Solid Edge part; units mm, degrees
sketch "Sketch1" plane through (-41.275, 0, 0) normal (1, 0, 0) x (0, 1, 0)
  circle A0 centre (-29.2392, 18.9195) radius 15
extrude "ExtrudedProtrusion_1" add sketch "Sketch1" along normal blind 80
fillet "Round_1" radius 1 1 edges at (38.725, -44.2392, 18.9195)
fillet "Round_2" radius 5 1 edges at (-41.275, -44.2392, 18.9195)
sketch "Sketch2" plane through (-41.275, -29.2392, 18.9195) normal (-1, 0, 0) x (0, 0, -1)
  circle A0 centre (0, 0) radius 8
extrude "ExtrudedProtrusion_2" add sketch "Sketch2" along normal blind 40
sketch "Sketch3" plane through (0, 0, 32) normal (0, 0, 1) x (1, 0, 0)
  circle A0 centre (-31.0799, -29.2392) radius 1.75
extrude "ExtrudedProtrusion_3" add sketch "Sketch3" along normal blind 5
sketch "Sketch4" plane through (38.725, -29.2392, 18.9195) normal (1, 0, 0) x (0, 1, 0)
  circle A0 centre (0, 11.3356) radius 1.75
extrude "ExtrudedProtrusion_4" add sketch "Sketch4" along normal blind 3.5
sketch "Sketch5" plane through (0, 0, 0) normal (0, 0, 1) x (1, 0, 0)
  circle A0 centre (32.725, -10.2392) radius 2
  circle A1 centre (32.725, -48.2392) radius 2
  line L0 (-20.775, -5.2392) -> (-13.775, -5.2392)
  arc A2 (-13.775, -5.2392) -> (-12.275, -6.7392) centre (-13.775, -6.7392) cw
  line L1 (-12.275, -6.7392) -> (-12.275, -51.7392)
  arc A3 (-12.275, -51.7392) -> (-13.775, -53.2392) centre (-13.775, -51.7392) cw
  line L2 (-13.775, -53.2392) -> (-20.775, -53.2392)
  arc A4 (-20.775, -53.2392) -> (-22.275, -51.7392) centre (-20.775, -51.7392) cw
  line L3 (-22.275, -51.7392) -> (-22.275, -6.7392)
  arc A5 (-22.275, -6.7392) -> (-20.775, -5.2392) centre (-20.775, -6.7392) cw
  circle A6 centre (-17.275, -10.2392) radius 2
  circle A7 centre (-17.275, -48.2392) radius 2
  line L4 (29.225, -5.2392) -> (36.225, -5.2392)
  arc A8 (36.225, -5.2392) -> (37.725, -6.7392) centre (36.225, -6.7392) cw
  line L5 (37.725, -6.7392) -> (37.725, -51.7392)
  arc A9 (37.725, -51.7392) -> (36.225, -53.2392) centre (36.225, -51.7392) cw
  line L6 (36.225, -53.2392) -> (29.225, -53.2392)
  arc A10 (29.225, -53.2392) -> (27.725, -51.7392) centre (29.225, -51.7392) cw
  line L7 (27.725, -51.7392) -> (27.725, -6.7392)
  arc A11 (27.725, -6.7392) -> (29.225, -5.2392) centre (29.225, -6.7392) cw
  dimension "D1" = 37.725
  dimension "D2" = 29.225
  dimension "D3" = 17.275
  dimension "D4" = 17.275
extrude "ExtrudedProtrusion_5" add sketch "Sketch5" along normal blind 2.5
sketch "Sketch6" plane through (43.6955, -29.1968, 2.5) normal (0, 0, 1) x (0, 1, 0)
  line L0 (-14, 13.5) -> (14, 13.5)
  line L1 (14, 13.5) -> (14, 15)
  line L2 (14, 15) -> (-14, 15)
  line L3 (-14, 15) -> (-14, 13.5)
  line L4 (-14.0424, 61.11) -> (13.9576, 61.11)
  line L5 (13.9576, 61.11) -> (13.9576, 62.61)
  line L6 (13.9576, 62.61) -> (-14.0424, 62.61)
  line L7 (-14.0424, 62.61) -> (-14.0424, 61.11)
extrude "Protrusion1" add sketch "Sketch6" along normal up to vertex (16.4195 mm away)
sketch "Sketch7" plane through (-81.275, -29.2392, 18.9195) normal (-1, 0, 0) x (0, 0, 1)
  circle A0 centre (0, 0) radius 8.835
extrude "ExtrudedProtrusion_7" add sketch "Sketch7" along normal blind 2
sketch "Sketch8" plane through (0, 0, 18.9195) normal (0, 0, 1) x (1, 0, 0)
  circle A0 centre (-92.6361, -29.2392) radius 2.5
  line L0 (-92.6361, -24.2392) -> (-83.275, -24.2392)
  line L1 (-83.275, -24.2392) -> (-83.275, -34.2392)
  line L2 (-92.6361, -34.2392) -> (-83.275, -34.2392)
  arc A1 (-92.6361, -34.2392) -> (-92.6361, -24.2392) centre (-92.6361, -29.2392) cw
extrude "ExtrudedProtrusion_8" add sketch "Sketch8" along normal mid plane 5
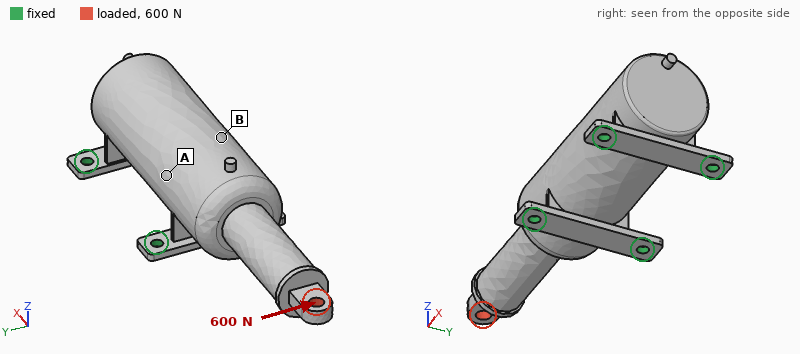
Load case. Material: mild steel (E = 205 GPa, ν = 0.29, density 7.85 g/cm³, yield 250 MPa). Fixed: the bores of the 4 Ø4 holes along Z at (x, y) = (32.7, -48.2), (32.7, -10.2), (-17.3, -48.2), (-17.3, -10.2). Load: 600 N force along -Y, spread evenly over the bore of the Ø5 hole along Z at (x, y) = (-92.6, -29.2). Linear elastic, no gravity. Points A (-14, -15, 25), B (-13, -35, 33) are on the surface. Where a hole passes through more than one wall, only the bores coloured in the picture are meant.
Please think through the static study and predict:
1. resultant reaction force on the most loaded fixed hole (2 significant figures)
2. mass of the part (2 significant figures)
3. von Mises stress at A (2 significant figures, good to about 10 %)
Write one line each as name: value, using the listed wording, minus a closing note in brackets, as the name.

resultant reaction force on the most loaded fixed hole: 810 N
mass of the part: 530 g
von Mises stress at A: 14 MPa
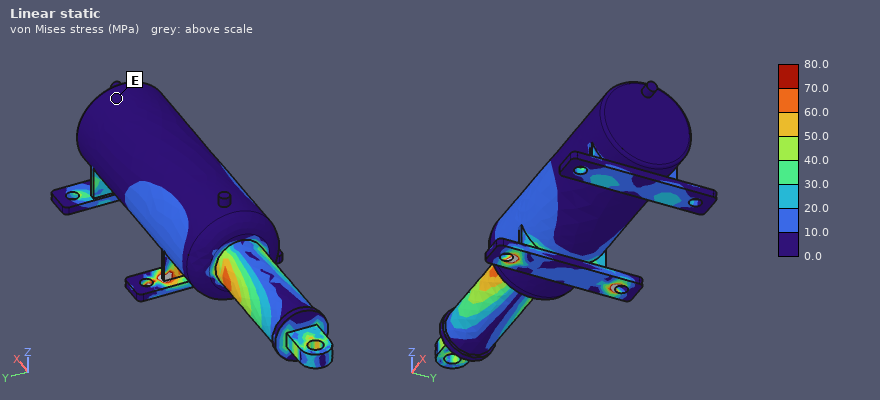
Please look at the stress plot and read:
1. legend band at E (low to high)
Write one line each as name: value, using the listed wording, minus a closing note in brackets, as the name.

legend band at E: 0.0 to 10.0 MPa
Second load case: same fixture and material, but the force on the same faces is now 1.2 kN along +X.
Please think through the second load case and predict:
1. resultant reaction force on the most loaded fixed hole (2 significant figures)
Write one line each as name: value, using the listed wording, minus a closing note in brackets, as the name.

resultant reaction force on the most loaded fixed hole: 400 N
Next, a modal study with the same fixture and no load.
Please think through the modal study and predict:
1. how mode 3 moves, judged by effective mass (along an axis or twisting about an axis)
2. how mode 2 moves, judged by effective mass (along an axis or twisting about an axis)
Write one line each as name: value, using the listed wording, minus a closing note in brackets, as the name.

how mode 3 moves, judged by effective mass: along X
how mode 2 moves, judged by effective mass: along Y
